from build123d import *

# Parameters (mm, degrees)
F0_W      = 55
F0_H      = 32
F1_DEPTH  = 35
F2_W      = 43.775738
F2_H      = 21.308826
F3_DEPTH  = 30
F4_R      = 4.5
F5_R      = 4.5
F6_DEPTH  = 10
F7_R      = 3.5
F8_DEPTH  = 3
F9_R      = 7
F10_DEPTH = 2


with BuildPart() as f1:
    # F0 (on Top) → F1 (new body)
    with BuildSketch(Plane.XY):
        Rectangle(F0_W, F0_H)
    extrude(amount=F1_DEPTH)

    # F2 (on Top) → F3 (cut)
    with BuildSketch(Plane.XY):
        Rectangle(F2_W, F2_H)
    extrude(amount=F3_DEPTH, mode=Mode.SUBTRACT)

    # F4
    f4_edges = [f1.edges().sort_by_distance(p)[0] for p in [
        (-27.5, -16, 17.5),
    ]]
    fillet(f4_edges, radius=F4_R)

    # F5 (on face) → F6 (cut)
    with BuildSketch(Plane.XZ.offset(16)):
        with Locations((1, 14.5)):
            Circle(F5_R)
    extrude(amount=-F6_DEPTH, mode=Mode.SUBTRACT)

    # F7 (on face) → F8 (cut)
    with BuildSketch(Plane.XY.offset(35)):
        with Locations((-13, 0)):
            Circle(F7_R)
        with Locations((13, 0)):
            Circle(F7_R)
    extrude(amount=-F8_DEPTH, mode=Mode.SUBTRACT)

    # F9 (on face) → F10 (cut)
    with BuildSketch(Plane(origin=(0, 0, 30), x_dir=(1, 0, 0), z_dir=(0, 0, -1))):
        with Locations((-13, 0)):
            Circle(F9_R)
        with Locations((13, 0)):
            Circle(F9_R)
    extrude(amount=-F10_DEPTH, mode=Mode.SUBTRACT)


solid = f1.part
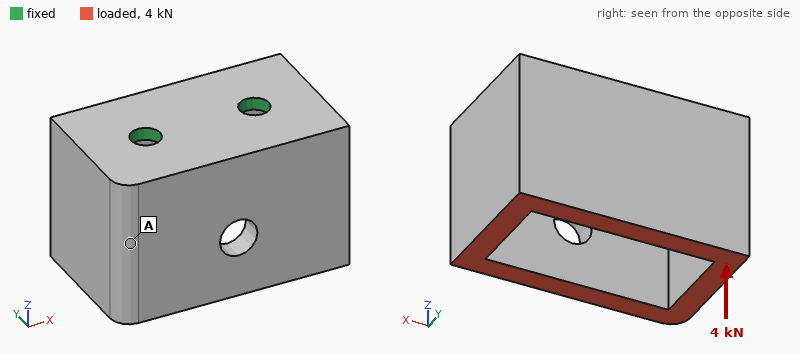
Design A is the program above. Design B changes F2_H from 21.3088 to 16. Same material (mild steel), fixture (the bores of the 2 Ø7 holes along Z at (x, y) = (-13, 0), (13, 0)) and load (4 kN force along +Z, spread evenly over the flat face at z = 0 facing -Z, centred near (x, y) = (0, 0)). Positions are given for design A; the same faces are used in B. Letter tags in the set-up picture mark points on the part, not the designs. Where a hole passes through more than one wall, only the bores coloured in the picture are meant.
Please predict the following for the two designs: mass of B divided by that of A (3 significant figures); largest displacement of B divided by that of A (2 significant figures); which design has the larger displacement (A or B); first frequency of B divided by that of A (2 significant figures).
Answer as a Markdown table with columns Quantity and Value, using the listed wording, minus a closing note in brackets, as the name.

| Quantity | Value |
|---|---|
| mass of B divided by that of A | 1.21 |
| largest displacement of B divided by that of A | 0.72 |
| which design has the larger displacement | A |
| first frequency of B divided by that of A | 0.95 |
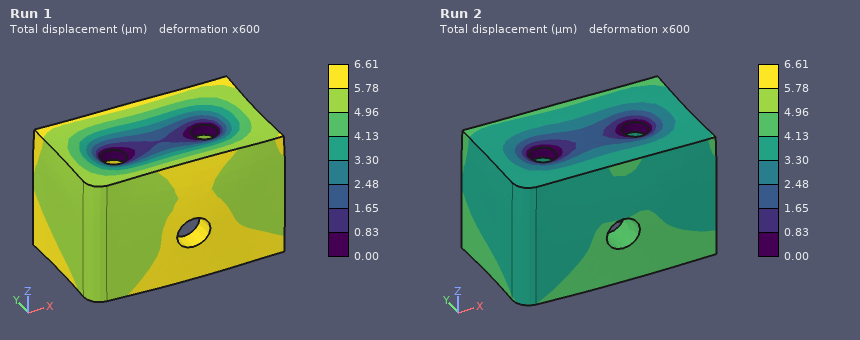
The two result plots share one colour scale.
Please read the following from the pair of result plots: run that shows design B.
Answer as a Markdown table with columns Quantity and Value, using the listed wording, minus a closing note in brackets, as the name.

| Quantity | Value |
|---|---|
| run that shows design B | Run 2 |
